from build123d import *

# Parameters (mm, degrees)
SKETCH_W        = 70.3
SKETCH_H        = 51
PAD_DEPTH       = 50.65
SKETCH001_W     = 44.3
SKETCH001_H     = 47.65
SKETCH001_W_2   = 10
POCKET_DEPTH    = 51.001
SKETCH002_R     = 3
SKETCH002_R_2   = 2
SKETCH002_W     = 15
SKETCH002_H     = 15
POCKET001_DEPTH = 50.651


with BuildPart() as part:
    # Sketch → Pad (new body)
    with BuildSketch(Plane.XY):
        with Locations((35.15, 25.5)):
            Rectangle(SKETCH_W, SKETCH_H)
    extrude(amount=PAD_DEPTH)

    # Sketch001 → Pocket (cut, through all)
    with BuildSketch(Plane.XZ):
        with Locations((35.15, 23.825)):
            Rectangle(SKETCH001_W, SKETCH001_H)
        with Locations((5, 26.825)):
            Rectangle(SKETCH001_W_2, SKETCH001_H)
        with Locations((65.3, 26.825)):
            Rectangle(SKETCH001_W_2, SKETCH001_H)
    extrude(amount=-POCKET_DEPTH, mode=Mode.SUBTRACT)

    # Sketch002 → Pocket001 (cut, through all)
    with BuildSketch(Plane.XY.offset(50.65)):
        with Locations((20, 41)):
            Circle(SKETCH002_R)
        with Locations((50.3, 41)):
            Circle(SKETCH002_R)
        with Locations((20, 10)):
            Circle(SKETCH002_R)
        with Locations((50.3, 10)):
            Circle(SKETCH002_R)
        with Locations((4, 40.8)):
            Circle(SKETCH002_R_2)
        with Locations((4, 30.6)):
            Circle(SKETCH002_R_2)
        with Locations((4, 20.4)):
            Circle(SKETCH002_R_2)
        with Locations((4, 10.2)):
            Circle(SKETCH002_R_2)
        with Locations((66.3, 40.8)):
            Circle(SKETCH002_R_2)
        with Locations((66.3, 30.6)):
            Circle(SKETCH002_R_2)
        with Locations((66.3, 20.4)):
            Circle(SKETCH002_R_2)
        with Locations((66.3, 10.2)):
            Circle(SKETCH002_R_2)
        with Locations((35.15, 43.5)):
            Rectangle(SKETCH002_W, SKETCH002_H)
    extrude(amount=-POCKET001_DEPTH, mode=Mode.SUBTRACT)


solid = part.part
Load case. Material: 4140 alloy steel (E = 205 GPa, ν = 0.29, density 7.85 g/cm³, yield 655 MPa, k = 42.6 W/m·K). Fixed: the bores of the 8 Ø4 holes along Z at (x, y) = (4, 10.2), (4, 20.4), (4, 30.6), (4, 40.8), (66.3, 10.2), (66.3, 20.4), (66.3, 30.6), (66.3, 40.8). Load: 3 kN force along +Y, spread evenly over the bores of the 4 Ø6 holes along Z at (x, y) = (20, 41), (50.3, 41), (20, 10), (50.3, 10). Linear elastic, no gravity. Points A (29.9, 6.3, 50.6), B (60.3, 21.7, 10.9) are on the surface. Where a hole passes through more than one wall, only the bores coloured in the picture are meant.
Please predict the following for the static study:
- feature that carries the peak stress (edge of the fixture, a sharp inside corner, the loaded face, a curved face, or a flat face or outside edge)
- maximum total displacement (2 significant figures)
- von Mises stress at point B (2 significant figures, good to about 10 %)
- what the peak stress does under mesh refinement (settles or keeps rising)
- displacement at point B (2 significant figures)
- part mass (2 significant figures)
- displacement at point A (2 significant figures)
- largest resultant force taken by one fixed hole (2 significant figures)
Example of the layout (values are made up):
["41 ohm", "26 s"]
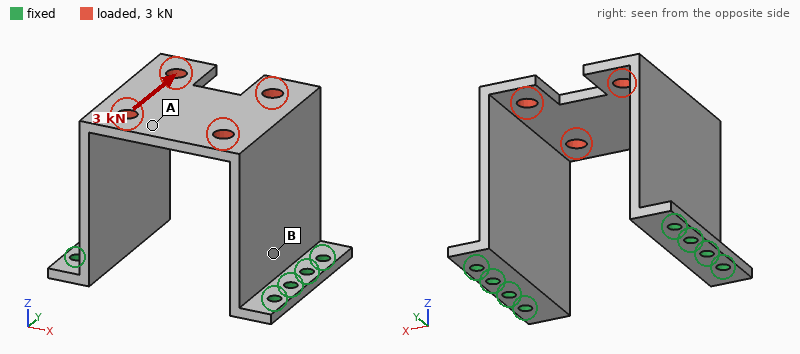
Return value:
["edge of the fixture", "96 µm", "59 MPa", "keeps rising", "19 µm", "190 g", "91 µm", "2.0 kN"]
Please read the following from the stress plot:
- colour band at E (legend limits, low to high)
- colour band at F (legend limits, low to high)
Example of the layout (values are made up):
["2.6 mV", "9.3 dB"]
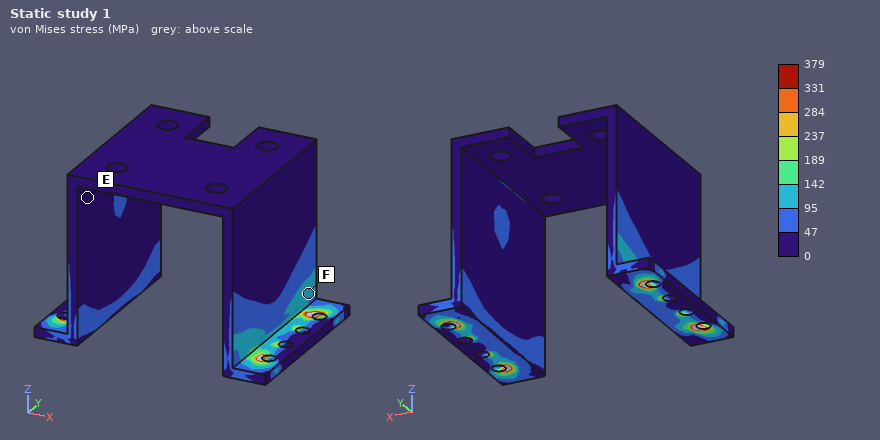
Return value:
["0 to 47 MPa", "95 to 142 MPa"]
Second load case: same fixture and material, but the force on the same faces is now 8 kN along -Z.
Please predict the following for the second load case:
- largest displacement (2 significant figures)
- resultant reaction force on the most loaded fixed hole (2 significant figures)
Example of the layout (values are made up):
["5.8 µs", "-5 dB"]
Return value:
["0.24 mm", "1.2 kN"]
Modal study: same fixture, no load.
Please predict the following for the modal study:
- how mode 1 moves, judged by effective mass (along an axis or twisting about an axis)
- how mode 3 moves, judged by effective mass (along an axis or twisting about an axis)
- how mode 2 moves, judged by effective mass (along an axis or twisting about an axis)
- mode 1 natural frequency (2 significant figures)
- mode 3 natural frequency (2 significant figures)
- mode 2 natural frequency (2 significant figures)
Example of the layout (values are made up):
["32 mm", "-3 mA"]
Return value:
["along X", "along Y", "twisting about Z", "930 Hz", "3000 Hz", "2800 Hz"]
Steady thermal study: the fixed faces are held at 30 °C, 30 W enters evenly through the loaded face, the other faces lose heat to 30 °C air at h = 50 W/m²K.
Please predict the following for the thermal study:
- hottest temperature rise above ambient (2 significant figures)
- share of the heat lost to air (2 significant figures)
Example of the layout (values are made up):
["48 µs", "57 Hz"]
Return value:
["67 K", "75 %"]
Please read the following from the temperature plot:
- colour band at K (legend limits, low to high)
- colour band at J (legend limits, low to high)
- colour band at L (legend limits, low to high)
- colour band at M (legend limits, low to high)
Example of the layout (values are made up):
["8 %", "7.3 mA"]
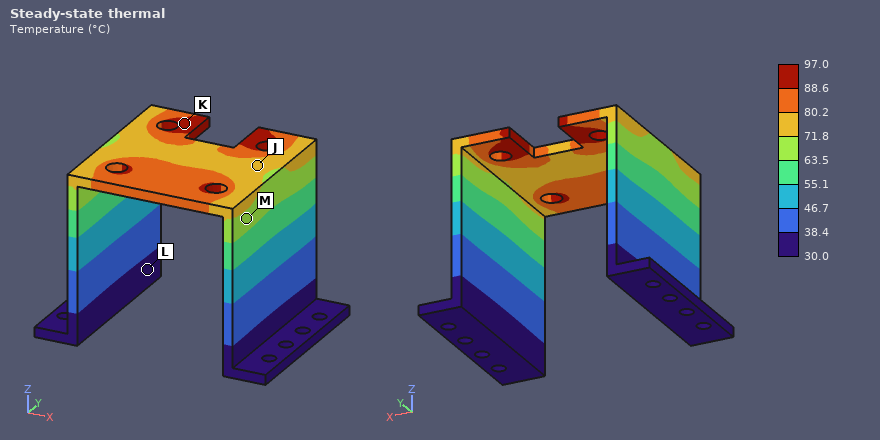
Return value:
["88.6 to 97.0 °C", "71.8 to 80.2 °C", "30.0 to 38.4 °C", "63.5 to 71.8 °C"]
